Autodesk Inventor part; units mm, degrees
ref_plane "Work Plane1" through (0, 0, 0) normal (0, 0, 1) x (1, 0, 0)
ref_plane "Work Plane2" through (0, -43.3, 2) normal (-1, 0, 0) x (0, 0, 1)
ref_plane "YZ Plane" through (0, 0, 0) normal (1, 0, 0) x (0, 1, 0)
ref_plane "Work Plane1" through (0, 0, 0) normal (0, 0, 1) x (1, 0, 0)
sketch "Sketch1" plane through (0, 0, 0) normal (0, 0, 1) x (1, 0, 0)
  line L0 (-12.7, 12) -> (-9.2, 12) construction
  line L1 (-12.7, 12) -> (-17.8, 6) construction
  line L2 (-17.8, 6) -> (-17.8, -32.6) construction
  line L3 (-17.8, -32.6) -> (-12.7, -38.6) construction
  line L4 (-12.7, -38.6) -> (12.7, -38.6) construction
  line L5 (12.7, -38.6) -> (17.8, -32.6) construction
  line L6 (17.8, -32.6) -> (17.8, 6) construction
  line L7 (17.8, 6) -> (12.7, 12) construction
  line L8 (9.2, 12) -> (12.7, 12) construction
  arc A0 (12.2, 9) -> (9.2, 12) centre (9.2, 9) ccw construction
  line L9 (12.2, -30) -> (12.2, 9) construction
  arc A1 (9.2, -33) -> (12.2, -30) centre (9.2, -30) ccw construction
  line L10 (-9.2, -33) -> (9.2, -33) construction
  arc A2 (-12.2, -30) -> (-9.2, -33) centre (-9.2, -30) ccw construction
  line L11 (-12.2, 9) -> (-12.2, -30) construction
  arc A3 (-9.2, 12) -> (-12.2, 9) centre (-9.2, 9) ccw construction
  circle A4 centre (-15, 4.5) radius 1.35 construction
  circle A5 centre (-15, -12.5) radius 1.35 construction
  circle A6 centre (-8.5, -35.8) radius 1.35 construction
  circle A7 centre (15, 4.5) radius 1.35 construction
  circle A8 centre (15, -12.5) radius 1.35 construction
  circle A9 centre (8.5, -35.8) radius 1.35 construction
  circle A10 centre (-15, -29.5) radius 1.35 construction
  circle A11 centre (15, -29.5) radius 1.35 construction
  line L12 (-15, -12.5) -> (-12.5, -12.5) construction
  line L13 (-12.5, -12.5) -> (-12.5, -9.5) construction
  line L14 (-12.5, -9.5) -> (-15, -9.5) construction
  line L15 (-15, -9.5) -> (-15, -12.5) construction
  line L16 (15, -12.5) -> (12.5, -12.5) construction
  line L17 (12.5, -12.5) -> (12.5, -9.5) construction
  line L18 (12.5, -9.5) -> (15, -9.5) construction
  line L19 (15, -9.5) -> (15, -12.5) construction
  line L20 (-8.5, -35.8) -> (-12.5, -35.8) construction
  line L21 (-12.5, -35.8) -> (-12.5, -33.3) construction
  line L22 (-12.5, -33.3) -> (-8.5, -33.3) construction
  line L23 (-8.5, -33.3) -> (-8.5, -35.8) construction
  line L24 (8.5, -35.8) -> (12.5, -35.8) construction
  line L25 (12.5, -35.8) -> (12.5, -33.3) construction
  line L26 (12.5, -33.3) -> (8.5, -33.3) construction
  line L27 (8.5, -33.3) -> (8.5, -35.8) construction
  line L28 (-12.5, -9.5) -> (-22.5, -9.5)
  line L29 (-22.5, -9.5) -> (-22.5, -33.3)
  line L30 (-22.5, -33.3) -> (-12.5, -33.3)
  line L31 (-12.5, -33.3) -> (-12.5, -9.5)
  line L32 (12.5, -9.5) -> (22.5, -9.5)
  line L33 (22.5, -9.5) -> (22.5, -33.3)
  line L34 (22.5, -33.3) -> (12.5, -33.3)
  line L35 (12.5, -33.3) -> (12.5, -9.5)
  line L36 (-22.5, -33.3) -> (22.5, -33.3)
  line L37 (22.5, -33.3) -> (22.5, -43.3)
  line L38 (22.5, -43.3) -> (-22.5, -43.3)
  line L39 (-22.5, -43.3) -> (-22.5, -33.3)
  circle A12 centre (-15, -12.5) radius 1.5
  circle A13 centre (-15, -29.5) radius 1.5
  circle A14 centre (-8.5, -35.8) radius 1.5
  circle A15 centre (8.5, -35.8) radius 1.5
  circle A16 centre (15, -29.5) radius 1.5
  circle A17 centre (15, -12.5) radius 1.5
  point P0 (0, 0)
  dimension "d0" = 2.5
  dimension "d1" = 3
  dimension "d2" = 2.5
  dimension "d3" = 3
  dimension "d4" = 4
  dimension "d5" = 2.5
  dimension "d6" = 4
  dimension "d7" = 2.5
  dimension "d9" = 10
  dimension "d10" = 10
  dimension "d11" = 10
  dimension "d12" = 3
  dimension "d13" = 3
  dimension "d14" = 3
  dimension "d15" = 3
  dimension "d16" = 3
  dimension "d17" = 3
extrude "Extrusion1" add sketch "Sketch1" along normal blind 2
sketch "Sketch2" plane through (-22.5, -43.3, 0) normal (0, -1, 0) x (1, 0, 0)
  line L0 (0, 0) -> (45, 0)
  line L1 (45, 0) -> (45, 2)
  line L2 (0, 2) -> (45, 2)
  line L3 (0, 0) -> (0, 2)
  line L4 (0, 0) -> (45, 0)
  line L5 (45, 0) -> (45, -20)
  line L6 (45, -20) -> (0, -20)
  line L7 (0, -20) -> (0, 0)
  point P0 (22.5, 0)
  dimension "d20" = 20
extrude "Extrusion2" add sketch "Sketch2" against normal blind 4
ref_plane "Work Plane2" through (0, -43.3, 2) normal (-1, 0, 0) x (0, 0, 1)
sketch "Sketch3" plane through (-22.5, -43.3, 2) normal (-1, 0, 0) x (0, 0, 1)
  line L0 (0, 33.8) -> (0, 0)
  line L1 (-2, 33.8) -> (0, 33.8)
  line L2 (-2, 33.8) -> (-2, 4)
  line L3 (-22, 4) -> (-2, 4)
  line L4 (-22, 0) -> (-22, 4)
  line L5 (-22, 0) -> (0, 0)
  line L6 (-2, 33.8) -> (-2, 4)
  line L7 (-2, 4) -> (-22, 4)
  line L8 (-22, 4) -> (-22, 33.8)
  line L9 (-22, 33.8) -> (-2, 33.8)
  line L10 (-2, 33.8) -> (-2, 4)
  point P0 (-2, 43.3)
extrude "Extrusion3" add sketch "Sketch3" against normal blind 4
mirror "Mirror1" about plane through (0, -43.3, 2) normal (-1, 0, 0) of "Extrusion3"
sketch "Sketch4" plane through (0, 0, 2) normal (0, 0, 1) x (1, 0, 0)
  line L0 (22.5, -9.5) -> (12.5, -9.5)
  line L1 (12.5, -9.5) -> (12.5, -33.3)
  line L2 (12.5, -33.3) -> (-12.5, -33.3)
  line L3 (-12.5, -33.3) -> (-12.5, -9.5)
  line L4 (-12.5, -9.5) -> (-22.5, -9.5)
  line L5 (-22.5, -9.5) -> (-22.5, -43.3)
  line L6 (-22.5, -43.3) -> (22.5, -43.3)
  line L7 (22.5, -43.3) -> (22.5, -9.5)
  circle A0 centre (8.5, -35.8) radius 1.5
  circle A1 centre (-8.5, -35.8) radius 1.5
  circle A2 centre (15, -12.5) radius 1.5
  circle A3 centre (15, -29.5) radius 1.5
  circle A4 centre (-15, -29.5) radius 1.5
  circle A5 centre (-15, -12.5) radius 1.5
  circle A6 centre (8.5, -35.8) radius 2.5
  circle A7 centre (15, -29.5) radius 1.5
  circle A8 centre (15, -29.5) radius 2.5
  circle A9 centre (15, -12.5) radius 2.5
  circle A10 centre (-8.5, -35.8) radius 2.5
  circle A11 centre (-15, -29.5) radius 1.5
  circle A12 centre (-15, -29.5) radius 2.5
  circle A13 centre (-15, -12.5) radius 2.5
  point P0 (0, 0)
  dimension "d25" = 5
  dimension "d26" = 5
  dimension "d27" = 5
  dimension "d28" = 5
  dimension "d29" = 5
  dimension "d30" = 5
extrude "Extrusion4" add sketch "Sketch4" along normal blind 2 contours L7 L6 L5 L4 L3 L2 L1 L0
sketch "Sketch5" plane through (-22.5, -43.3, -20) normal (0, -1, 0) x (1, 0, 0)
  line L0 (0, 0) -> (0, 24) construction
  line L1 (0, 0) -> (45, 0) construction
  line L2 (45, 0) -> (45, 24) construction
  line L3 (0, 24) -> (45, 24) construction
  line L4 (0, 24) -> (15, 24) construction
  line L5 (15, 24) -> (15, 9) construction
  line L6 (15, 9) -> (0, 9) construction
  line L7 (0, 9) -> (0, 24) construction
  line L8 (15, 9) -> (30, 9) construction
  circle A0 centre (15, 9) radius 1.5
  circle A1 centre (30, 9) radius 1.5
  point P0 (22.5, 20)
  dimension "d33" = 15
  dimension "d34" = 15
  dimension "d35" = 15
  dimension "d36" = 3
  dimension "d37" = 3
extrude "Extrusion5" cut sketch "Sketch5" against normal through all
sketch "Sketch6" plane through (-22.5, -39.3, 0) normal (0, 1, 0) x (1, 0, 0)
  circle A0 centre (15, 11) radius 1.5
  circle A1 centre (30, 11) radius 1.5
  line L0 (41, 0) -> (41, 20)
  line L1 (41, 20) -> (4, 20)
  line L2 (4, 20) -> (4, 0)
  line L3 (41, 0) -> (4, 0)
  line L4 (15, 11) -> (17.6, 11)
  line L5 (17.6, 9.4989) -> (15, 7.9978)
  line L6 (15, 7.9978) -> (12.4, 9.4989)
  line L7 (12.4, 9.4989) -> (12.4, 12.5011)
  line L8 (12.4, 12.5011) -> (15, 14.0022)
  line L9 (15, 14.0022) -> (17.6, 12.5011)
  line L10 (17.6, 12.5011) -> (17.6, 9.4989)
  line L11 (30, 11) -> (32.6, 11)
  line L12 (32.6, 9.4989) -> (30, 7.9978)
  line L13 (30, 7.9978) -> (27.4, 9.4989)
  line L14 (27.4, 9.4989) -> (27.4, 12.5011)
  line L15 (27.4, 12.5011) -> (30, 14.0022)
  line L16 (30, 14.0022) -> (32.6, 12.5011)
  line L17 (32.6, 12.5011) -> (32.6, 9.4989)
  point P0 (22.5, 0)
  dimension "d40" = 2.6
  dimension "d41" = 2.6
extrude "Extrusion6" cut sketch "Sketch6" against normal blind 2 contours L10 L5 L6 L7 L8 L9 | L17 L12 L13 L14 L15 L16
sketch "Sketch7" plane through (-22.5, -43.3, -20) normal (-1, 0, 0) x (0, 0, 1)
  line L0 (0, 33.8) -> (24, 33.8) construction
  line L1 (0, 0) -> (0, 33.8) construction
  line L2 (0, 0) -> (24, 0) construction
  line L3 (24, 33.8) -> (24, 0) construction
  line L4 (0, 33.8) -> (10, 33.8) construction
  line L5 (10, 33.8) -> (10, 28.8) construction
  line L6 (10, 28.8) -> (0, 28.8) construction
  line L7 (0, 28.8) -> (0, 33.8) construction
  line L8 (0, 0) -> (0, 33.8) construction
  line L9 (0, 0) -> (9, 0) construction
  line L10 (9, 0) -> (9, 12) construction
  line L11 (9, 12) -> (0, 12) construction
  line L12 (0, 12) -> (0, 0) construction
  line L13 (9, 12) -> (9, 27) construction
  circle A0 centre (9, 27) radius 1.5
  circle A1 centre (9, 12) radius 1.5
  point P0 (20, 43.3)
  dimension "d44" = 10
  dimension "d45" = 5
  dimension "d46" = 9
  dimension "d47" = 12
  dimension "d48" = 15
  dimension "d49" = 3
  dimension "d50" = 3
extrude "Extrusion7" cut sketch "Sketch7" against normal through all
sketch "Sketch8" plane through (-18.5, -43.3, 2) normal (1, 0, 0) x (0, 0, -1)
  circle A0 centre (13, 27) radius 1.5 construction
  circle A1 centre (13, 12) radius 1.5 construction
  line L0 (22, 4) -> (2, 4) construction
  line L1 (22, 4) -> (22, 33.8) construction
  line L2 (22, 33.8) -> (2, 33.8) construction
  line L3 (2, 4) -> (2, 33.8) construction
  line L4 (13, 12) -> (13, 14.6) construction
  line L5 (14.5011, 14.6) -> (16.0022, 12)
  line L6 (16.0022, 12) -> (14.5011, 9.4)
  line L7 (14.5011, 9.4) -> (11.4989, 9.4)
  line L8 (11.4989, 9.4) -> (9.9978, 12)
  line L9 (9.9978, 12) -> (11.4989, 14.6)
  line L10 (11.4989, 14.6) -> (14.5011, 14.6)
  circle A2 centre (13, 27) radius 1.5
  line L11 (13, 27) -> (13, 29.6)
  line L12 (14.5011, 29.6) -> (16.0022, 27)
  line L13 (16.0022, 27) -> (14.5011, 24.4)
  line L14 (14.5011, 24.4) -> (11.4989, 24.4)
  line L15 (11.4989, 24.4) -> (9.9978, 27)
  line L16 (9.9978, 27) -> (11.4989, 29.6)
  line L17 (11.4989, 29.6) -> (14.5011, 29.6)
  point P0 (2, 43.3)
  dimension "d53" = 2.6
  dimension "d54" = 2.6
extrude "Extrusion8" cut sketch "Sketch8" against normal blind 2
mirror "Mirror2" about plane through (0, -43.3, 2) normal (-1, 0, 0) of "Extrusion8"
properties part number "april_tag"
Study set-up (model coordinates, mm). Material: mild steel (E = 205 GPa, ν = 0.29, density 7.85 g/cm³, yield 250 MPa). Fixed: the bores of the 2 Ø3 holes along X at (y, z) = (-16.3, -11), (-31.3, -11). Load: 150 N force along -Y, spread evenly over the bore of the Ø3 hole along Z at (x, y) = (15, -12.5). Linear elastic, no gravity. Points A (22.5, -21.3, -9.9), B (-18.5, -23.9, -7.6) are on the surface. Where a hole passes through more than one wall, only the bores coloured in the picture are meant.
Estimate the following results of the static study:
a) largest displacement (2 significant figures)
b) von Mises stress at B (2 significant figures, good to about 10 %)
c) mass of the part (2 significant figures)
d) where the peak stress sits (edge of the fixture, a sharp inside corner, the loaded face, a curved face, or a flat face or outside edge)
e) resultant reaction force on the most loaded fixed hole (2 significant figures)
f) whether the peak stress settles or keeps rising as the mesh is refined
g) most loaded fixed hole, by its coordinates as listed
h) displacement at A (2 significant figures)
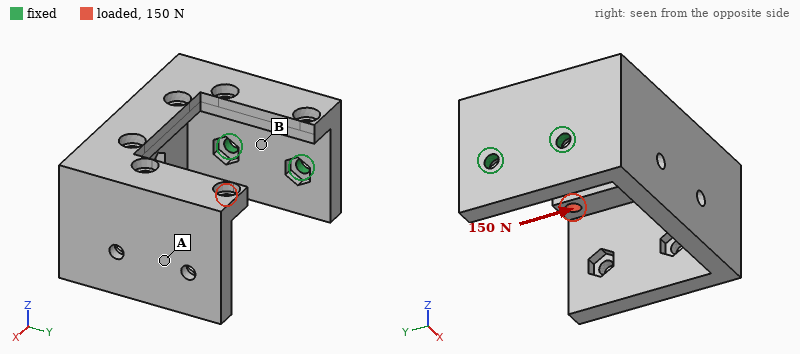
0.10 mm
29 MPa
89 g
a sharp inside corner
400 N
keeps rising
(-16.3, -11)
0.090 mm
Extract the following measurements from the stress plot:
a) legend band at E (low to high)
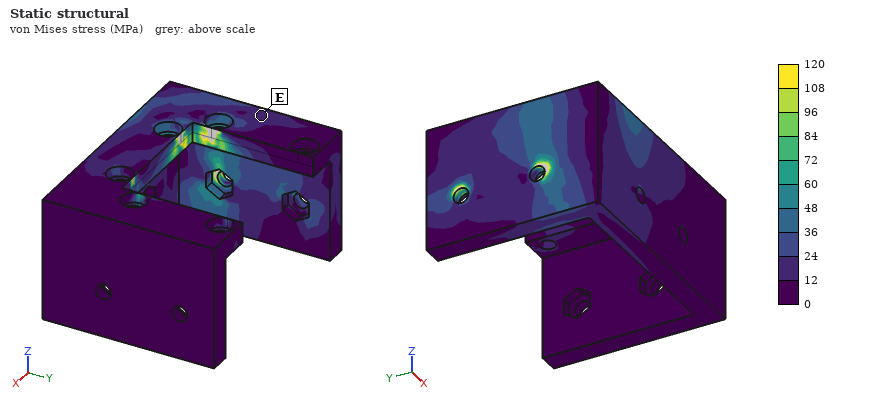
12 to 24 MPa
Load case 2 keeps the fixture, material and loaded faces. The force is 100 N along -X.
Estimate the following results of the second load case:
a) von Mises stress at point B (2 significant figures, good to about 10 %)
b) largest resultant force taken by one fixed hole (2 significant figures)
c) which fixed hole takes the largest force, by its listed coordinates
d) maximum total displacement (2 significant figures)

14 MPa
120 N
(-16.3, -11)
73 µm
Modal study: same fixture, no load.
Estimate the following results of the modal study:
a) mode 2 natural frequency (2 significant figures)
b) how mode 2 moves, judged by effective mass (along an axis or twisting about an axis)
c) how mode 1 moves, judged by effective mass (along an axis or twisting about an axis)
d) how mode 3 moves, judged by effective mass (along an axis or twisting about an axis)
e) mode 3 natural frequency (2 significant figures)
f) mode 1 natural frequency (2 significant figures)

990 Hz
along Y
along Z
along X
2400 Hz
810 Hz
